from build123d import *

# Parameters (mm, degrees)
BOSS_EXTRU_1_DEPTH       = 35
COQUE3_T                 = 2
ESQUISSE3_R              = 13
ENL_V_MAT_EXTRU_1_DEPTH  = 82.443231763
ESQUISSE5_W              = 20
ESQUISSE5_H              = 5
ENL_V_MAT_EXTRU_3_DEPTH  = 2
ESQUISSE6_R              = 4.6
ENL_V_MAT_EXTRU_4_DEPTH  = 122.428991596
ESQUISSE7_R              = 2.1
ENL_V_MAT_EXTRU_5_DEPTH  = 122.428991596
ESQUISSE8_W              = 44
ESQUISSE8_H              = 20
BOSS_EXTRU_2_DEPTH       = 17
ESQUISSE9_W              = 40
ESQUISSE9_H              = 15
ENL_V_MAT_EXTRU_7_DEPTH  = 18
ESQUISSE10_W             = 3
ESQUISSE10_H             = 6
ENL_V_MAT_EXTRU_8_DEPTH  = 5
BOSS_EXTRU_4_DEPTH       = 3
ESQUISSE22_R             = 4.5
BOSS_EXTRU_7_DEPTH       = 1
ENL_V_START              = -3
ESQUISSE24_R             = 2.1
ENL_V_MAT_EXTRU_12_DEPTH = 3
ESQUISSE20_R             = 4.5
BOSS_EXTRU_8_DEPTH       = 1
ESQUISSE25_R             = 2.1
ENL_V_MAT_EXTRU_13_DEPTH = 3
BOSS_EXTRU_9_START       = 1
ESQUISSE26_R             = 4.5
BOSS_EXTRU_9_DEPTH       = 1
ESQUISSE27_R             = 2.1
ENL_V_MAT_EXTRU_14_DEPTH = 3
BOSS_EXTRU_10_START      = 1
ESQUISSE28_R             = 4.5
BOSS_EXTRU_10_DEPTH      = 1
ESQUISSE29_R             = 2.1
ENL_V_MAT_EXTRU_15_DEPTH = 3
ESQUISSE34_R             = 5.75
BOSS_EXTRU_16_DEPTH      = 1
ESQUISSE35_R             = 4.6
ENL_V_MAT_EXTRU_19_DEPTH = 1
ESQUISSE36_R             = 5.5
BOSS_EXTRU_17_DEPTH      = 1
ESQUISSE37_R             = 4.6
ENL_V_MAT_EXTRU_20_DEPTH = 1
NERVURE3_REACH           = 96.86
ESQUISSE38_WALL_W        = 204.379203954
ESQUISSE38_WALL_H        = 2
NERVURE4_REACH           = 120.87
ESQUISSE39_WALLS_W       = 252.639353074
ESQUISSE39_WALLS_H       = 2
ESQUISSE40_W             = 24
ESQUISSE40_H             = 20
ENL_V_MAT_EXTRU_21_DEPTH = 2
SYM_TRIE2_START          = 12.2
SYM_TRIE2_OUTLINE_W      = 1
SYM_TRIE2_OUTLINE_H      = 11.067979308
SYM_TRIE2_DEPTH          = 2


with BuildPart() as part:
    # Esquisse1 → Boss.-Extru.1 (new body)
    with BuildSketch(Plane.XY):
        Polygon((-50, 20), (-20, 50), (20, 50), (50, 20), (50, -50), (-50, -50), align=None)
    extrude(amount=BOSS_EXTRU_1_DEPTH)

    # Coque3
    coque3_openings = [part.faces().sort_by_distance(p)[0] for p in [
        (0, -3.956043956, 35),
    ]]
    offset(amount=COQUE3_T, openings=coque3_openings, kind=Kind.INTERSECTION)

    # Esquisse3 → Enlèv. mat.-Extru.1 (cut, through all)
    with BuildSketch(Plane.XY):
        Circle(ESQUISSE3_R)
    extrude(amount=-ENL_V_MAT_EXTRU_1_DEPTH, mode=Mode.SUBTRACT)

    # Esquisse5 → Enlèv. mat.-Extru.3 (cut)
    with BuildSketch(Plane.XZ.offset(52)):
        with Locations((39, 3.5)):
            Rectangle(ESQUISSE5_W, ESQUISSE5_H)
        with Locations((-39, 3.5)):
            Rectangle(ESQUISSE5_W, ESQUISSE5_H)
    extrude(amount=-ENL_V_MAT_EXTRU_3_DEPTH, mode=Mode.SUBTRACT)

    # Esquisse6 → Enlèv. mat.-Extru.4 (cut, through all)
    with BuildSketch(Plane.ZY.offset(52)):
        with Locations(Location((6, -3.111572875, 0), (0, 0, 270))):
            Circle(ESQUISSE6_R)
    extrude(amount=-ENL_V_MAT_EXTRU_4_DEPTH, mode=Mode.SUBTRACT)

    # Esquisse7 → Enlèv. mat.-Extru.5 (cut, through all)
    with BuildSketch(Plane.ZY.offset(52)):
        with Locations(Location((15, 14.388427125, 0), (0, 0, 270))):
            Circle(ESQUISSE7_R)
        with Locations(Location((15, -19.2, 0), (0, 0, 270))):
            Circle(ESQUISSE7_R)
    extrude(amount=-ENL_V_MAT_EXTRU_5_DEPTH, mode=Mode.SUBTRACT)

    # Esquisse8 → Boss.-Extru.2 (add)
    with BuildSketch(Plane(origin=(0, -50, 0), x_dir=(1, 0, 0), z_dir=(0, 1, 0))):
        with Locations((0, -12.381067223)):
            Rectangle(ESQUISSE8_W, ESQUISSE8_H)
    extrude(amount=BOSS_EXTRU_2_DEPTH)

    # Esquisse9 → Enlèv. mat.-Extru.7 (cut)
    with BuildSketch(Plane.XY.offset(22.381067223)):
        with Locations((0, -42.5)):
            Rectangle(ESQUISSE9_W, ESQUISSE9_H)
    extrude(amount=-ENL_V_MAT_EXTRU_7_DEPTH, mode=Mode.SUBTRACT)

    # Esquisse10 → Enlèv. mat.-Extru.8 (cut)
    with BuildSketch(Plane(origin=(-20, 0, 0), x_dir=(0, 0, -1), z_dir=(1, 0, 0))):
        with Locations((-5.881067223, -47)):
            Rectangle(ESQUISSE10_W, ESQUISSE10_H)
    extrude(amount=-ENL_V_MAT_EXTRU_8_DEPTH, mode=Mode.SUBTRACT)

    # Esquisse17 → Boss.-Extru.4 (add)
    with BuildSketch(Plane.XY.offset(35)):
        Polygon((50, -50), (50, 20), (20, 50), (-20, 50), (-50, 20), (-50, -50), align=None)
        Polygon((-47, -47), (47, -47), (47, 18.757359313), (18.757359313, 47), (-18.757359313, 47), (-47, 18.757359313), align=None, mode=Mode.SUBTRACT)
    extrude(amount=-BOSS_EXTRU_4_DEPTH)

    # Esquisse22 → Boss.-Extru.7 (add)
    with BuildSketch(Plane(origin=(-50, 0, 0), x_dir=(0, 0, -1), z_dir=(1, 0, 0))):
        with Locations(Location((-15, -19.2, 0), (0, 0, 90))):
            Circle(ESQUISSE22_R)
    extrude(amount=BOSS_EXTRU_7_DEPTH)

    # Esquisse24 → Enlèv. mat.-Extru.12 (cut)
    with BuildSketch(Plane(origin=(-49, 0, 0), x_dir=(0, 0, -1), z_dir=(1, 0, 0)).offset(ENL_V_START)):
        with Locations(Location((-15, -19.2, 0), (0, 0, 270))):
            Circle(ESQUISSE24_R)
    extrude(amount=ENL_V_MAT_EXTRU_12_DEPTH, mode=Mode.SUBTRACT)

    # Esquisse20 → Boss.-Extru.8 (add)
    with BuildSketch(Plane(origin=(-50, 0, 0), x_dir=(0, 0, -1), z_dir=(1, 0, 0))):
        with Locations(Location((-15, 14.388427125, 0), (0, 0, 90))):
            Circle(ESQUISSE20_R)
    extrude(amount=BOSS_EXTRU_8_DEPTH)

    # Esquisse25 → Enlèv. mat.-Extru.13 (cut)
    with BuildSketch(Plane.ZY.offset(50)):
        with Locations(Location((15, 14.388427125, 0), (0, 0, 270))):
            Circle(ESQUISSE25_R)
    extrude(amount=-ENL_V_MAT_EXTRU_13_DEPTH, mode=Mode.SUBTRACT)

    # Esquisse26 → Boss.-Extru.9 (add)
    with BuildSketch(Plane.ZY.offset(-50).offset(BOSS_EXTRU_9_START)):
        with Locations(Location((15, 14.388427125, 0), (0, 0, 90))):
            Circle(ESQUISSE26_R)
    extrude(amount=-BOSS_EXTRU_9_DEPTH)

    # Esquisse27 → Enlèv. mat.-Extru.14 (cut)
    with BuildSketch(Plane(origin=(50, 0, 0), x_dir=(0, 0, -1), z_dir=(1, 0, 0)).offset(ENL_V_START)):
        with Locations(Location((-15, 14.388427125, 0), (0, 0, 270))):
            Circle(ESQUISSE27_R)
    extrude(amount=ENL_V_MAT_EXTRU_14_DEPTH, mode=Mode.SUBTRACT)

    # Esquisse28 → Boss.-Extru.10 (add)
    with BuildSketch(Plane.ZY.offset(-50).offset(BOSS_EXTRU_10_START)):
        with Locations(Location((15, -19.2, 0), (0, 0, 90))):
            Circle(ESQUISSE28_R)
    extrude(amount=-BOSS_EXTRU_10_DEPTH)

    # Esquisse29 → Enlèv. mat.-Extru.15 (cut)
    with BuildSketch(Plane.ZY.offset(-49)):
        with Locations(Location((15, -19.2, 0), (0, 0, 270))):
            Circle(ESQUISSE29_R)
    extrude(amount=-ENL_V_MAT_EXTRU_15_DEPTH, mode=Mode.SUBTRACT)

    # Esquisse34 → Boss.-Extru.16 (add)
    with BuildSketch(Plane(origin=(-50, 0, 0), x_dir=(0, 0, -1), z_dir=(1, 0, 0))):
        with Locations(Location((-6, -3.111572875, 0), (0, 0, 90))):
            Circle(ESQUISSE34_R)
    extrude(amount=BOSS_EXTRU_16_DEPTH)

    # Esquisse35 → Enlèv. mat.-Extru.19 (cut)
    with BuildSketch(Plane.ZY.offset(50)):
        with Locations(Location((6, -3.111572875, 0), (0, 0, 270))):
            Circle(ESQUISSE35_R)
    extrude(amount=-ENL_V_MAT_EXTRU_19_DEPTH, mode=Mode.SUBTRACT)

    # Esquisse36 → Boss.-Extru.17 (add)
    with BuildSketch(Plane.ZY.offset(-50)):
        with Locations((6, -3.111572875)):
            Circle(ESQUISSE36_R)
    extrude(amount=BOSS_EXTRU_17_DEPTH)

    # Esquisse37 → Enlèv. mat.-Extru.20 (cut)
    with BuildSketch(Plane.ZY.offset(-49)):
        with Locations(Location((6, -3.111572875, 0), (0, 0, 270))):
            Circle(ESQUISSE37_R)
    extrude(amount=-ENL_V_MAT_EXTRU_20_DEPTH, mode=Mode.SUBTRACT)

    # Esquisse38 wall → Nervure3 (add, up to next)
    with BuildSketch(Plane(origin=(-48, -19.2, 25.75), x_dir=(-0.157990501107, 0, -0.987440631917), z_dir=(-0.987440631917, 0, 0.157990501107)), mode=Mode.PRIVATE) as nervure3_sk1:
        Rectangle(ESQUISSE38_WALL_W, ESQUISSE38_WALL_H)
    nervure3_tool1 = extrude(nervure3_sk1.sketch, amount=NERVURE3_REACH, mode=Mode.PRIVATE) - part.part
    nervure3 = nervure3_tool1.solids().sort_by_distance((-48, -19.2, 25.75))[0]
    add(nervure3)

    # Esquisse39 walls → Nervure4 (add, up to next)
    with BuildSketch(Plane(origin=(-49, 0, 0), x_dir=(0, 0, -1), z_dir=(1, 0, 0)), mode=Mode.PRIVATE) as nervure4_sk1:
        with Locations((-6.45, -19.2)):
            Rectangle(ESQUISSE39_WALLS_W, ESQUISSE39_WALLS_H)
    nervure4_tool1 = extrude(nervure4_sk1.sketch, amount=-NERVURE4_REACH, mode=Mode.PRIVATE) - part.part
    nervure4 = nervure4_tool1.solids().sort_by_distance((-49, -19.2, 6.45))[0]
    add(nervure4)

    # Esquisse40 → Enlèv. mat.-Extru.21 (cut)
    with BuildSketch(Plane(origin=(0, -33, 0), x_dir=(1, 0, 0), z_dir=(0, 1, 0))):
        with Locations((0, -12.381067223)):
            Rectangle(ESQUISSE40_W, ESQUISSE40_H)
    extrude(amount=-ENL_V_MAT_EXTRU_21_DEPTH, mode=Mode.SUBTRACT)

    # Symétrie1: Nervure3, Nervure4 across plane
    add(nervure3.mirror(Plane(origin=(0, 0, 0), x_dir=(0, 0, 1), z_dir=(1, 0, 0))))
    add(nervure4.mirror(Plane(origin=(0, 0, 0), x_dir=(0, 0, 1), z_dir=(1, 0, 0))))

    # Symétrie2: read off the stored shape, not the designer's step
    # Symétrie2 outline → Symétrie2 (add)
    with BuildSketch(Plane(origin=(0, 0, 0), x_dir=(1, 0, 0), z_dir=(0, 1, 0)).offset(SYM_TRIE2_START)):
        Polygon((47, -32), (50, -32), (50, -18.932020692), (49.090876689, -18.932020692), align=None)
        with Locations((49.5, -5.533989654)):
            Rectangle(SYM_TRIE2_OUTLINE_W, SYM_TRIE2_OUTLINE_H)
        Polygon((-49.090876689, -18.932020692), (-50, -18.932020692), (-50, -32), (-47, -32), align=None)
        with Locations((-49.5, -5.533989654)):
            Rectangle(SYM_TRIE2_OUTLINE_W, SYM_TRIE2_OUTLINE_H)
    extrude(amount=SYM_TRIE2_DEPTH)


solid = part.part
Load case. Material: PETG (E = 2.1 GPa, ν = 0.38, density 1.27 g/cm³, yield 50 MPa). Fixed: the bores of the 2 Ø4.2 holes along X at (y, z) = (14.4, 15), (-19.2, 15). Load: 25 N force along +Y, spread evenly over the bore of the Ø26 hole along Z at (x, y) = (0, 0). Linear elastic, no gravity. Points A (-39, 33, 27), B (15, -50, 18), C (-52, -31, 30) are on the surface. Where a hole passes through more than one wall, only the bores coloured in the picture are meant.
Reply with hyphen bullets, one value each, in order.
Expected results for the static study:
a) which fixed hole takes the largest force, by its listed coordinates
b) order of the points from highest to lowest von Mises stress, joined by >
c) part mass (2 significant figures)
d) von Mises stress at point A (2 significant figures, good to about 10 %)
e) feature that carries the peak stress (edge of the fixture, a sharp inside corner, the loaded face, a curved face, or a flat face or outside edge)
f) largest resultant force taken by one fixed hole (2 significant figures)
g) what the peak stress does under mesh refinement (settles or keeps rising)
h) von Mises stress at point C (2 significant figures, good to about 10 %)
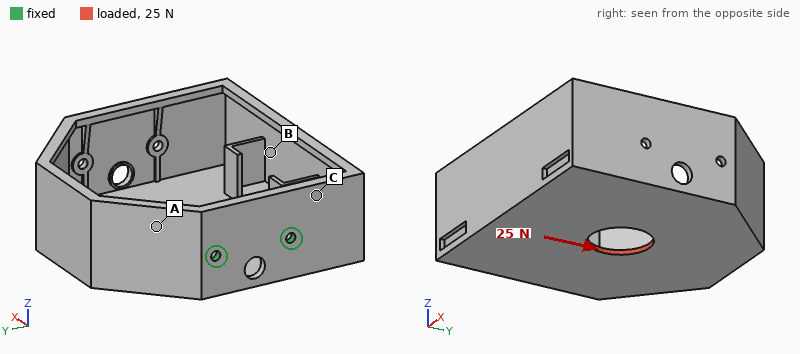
- (-19.2, 15)
- C > A > B
- 65 g
- 1.1 MPa
- edge of the fixture
- 38 N
- keeps rising
- 2.3 MPa
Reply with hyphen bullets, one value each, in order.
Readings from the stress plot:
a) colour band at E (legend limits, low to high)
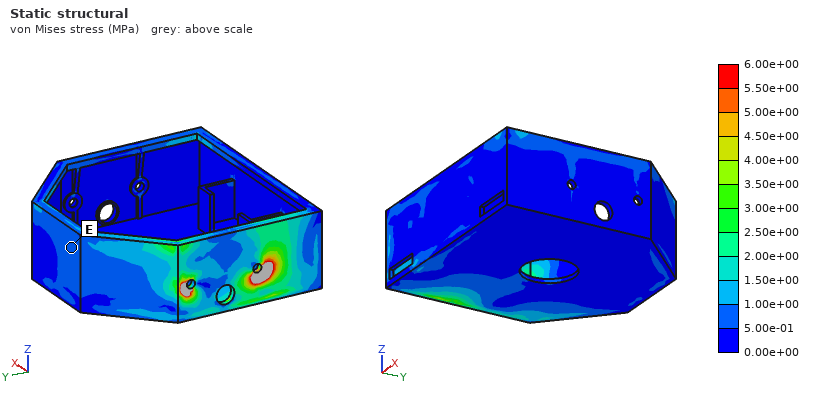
- 5.00e-01 to 1.00e+00 MPa
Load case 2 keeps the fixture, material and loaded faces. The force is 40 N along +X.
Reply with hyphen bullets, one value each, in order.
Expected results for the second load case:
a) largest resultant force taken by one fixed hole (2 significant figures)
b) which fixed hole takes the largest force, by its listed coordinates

- 24 N
- (14.4, 15)
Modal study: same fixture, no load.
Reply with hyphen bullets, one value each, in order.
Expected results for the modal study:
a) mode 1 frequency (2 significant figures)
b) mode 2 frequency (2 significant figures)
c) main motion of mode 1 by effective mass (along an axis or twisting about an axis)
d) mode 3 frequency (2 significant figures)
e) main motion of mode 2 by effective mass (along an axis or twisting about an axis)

- 48 Hz
- 86 Hz
- along Z
- 190 Hz
- along Y
